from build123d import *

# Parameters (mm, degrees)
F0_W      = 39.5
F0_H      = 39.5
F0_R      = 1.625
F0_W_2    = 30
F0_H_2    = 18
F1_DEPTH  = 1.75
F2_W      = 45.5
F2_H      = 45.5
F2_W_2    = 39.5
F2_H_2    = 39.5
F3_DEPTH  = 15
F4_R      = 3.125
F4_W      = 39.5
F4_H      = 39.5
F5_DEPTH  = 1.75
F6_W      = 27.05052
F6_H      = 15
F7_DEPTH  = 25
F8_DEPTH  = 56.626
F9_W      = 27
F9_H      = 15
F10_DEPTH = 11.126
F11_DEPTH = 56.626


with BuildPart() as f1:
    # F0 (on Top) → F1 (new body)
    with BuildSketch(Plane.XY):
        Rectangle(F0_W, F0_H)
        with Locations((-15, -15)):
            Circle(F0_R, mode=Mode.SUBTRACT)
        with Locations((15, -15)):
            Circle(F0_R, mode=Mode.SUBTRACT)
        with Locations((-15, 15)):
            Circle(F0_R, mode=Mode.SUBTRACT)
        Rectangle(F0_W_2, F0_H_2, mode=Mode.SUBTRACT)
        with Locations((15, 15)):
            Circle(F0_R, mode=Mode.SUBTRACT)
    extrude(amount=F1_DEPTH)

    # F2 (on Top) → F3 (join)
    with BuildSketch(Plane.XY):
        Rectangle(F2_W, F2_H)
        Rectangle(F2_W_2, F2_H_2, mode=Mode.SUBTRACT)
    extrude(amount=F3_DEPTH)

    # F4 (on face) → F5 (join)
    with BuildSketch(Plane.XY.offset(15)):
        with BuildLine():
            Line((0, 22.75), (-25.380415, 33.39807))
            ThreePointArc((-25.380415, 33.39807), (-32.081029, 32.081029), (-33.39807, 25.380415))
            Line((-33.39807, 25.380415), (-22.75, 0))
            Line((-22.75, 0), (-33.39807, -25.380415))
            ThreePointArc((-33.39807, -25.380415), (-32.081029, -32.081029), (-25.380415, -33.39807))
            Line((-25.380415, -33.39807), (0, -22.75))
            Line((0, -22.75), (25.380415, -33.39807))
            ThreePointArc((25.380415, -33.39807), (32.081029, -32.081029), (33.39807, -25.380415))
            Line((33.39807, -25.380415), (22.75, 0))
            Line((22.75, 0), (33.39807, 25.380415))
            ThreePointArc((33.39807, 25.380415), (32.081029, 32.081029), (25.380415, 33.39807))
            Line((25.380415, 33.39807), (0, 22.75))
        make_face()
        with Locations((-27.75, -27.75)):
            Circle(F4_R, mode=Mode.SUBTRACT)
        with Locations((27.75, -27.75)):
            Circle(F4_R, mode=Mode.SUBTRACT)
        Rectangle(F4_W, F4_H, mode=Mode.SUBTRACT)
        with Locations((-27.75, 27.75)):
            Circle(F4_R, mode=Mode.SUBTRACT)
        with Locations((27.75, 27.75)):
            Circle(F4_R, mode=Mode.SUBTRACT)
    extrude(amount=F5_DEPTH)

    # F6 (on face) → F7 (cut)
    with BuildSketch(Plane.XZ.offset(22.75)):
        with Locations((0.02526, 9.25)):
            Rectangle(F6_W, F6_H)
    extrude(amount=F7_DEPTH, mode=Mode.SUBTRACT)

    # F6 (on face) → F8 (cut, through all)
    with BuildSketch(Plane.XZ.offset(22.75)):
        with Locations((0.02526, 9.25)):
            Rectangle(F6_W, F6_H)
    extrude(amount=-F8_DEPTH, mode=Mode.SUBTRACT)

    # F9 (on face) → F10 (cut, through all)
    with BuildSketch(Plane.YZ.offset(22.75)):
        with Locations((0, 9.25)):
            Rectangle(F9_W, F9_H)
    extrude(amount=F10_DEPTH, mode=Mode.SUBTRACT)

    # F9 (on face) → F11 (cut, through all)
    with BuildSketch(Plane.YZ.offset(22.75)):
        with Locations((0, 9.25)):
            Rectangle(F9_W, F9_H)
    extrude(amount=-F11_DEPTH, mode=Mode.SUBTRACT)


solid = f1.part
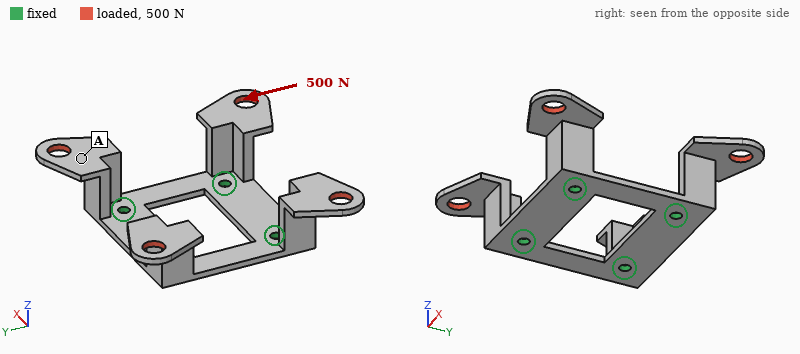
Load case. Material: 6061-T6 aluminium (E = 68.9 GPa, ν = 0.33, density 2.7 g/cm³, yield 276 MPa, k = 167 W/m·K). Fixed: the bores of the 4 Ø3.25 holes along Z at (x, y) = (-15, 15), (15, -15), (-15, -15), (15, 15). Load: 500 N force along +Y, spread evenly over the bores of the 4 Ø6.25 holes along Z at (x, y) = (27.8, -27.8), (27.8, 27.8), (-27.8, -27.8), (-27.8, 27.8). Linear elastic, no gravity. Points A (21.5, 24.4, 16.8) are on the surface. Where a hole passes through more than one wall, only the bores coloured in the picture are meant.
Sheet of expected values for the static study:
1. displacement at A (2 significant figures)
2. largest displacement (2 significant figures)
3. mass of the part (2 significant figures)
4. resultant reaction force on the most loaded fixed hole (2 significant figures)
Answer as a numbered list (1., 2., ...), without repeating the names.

1. 0.20 mm
2. 0.31 mm
3. 19 g
4. 130 N
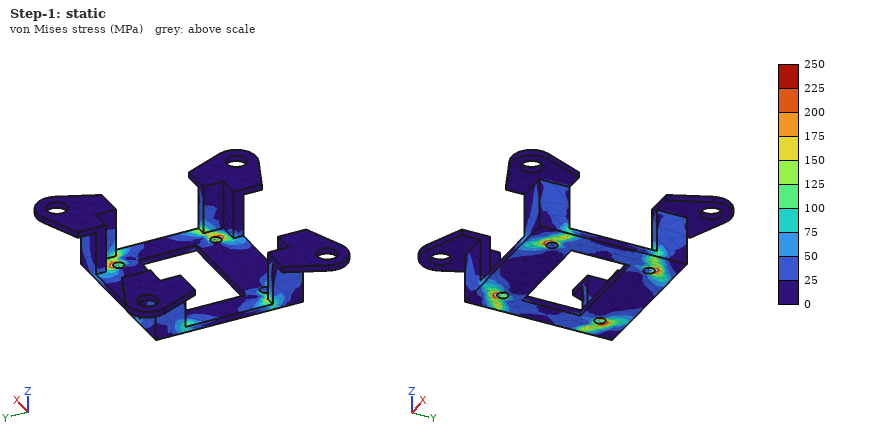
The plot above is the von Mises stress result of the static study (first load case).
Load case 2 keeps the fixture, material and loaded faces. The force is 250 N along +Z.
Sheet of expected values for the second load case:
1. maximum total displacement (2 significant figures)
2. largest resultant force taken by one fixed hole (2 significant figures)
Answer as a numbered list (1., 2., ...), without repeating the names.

1. 0.29 mm
2. 63 N
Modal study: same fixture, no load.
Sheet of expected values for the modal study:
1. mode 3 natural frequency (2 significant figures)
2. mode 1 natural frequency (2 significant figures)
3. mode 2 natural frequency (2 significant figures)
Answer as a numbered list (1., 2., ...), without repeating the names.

1. 2300 Hz
2. 2300 Hz
3. 2300 Hz
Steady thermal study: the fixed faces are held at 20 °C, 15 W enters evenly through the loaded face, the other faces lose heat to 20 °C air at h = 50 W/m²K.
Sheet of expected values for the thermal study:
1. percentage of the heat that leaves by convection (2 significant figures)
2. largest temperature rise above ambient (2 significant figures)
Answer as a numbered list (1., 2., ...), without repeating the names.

1. 18 %
2. 22 K
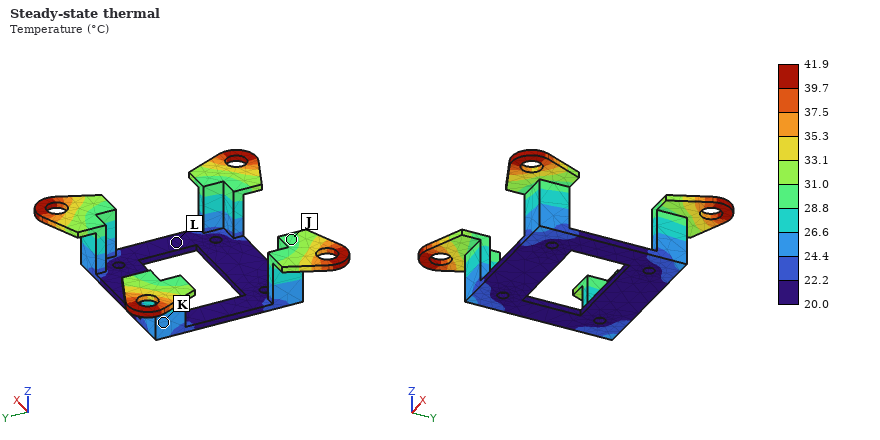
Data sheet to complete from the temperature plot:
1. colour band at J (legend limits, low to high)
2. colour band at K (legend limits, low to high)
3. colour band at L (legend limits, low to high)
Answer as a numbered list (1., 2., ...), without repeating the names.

1. 28.8 to 31.0 °C
2. 24.4 to 26.6 °C
3. 20.0 to 22.2 °C
